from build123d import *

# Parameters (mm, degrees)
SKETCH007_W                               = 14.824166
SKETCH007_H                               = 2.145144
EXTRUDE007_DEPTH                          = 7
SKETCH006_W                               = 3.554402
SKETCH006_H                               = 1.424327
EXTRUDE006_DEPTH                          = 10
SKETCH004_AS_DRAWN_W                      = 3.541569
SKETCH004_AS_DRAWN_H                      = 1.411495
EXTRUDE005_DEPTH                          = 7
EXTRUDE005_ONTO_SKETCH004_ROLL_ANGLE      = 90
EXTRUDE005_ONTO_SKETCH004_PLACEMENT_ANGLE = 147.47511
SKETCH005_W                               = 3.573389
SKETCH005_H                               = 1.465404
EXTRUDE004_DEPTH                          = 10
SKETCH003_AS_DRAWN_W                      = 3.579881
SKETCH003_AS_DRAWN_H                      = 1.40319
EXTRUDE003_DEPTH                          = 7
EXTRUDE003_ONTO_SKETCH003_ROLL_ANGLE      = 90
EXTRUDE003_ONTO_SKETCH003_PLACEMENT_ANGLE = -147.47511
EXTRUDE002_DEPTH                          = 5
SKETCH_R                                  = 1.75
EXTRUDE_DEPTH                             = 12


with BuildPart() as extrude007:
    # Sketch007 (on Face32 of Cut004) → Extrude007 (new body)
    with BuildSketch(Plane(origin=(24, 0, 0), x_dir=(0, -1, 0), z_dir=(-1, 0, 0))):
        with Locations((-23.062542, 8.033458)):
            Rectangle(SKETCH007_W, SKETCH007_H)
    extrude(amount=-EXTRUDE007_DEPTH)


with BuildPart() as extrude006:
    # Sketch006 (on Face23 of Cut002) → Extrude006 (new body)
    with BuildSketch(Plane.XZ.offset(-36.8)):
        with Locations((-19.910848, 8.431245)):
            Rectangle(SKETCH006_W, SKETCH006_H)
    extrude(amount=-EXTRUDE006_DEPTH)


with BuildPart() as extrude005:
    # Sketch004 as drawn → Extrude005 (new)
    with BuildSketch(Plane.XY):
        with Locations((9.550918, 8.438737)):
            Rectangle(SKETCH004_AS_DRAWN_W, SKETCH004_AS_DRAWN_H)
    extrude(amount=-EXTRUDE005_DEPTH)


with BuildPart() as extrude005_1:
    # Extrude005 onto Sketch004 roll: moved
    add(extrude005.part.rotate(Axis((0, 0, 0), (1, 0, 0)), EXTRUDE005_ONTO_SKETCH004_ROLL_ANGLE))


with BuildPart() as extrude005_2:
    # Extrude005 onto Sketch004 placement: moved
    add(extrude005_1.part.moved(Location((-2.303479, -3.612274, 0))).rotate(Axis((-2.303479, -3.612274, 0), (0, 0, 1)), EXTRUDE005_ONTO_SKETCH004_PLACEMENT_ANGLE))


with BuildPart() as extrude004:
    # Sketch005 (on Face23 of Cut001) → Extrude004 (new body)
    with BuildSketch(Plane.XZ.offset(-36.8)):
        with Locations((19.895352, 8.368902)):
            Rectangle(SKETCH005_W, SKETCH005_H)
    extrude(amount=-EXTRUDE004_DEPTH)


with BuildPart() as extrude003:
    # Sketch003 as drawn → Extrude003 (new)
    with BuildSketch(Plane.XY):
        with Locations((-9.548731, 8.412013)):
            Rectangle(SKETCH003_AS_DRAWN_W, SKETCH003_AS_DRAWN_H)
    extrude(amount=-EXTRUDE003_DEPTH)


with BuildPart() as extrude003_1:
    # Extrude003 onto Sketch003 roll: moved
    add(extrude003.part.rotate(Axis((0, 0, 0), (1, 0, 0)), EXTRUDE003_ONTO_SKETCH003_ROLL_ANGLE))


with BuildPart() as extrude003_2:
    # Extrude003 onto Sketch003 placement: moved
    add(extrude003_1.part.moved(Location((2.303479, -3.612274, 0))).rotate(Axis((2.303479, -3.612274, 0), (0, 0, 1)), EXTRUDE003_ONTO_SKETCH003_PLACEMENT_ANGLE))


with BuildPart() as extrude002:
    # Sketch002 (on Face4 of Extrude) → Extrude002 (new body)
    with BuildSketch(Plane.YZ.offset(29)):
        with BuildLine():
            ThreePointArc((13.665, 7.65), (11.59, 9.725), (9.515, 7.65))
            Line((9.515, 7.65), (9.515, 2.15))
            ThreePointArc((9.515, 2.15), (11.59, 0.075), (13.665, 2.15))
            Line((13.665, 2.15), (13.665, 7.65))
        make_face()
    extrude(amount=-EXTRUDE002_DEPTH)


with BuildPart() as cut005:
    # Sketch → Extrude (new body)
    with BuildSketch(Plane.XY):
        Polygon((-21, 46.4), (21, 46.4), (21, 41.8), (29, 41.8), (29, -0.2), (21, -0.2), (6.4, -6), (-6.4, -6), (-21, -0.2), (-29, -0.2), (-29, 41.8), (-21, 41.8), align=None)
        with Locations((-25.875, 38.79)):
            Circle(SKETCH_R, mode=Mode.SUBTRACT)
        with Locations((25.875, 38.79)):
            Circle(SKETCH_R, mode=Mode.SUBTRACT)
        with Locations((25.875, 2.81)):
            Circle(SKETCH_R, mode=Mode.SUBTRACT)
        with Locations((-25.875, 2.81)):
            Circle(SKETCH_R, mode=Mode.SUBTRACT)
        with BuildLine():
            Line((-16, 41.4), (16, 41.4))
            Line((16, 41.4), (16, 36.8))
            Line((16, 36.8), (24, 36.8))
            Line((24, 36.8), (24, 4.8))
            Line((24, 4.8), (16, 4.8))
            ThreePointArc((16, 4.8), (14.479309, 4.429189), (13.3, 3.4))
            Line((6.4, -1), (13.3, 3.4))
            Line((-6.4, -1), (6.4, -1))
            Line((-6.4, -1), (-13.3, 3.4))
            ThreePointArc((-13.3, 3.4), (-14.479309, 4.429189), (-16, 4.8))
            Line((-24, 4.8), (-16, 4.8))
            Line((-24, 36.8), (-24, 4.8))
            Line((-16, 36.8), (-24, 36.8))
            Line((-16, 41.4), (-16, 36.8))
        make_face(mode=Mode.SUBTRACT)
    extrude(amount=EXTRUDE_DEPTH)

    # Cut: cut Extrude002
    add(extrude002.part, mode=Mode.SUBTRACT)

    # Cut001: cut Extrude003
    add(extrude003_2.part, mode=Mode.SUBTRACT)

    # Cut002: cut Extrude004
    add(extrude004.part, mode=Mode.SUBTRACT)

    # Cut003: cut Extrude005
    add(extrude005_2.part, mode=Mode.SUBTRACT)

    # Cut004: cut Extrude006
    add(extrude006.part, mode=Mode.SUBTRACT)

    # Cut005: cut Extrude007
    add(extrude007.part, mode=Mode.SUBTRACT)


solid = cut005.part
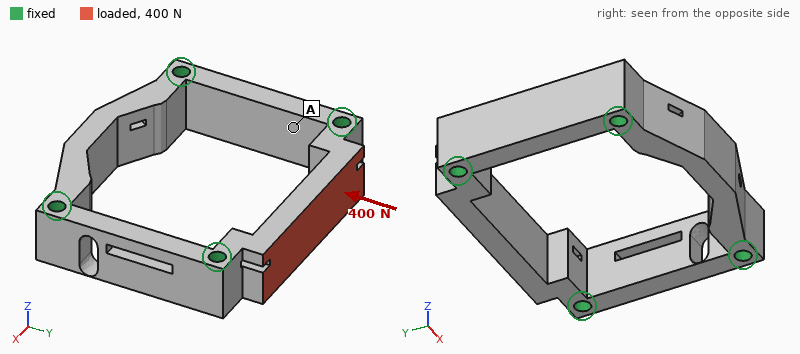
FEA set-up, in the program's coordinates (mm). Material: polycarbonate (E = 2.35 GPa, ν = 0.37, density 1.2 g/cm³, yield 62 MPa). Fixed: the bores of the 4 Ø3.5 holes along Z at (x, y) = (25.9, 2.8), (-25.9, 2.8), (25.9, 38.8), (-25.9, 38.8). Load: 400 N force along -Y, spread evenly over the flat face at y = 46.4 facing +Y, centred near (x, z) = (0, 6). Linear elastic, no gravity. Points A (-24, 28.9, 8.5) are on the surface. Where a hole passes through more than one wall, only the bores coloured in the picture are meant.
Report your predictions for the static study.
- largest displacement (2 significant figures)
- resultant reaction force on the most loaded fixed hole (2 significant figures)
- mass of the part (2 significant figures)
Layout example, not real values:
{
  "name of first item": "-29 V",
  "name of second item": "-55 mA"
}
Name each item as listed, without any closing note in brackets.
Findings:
{
  "largest displacement": "0.33 mm",
  "resultant reaction force on the most loaded fixed hole": "340 N",
  "mass of the part": "13 g"
}
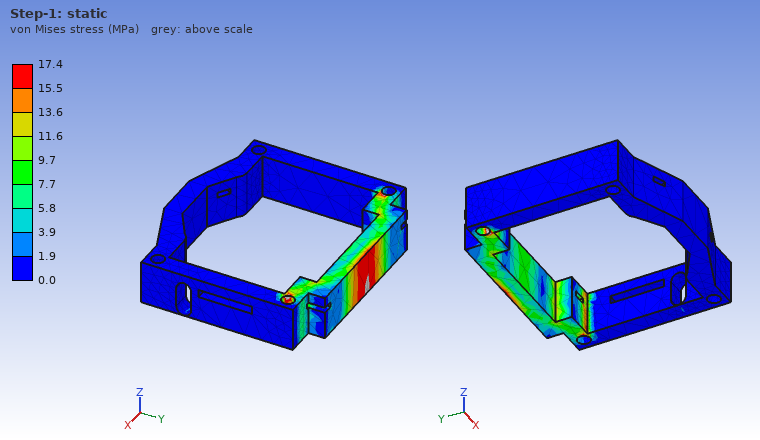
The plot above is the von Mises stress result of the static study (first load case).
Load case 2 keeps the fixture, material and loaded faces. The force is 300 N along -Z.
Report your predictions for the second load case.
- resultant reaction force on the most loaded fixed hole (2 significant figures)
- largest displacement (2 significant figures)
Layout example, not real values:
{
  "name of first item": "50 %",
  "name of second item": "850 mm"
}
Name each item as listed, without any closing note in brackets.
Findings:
{
  "resultant reaction force on the most loaded fixed hole": "150 N",
  "largest displacement": "0.24 mm"
}
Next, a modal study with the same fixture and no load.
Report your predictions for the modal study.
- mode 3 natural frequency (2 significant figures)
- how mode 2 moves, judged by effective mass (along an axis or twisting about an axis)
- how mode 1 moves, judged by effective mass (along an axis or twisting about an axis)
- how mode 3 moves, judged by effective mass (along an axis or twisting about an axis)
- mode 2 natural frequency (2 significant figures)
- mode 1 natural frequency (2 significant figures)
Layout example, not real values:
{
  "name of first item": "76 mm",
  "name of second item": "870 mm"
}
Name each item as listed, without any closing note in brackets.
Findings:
{
  "mode 3 natural frequency": "4400 Hz",
  "how mode 2 moves, judged by effective mass": "along Z",
  "how mode 1 moves, judged by effective mass": "along Y",
  "how mode 3 moves, judged by effective mass": "along Y",
  "mode 2 natural frequency": "4000 Hz",
  "mode 1 natural frequency": "3600 Hz"
}
